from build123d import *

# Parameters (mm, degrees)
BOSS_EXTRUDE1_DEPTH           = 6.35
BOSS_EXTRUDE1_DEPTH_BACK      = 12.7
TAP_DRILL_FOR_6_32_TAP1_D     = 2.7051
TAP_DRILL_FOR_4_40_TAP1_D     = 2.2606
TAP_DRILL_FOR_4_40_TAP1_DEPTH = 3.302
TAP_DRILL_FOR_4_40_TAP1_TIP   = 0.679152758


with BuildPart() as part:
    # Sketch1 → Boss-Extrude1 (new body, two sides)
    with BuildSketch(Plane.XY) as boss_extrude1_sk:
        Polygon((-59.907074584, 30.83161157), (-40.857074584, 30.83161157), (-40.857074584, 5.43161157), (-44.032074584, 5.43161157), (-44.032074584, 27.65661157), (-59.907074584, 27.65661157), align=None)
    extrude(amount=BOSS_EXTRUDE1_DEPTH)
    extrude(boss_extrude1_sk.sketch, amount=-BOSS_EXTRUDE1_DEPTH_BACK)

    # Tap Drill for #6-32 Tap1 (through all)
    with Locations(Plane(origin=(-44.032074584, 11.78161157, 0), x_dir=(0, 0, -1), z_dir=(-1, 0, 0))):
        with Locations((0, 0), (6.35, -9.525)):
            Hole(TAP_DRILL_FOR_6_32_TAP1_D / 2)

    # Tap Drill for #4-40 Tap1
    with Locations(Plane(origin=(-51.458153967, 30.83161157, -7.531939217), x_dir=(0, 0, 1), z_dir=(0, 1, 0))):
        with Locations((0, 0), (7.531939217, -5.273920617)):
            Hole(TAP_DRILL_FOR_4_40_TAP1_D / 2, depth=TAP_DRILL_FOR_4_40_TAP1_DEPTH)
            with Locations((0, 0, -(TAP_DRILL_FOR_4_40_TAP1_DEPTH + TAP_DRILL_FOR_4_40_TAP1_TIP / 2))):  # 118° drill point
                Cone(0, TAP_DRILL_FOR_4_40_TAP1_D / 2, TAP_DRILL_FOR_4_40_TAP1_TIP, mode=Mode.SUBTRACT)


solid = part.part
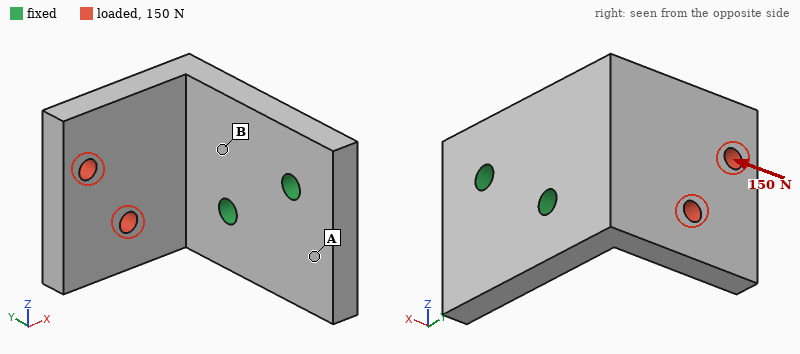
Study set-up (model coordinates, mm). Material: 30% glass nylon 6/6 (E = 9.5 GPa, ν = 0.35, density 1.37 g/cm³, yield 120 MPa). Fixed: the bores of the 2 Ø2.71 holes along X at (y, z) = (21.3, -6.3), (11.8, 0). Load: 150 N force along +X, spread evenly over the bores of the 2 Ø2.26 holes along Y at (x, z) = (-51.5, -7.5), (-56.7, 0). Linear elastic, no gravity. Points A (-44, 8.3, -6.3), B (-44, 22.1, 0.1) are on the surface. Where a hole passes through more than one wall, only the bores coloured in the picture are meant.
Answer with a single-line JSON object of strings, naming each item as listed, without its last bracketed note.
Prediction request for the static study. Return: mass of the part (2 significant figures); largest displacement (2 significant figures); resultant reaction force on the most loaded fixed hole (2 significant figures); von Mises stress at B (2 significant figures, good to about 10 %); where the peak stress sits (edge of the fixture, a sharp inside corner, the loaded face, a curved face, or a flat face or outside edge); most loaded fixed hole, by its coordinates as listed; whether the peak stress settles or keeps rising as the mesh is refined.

{"mass of the part": "3.3 g", "largest displacement": "0.25 mm", "resultant reaction force on the most loaded fixed hole": "170 N", "von Mises stress at B": "18 MPa", "where the peak stress sits": "edge of the fixture", "most loaded fixed hole, by its coordinates as listed": "(21.3, -6.3)", "whether the peak stress settles or keeps rising as the mesh is refined": "keeps rising"}
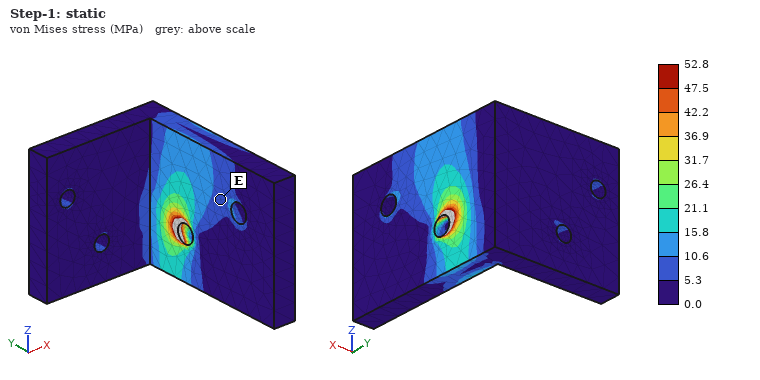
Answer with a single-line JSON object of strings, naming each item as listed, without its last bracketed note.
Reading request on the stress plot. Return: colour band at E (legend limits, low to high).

{"colour band at E": "5.3 to 10.6 MPa"}
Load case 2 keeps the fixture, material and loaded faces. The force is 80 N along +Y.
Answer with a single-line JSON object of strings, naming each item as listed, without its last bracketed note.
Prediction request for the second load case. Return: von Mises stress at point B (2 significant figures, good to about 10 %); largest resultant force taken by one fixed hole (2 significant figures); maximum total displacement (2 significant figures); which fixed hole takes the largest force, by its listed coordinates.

{"von Mises stress at point B": "20 MPa", "largest resultant force taken by one fixed hole": "66 N", "maximum total displacement": "0.42 mm", "which fixed hole takes the largest force, by its listed coordinates": "(21.3, -6.3)"}
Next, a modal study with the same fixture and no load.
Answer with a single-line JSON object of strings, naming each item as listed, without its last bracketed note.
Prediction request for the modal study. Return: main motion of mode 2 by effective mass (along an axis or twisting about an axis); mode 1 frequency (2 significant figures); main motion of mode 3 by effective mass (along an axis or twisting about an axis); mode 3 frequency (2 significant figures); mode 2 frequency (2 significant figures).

{"main motion of mode 2 by effective mass": "along Z", "mode 1 frequency": "2500 Hz", "main motion of mode 3 by effective mass": "along X", "mode 3 frequency": "7800 Hz", "mode 2 frequency": "3500 Hz"}
